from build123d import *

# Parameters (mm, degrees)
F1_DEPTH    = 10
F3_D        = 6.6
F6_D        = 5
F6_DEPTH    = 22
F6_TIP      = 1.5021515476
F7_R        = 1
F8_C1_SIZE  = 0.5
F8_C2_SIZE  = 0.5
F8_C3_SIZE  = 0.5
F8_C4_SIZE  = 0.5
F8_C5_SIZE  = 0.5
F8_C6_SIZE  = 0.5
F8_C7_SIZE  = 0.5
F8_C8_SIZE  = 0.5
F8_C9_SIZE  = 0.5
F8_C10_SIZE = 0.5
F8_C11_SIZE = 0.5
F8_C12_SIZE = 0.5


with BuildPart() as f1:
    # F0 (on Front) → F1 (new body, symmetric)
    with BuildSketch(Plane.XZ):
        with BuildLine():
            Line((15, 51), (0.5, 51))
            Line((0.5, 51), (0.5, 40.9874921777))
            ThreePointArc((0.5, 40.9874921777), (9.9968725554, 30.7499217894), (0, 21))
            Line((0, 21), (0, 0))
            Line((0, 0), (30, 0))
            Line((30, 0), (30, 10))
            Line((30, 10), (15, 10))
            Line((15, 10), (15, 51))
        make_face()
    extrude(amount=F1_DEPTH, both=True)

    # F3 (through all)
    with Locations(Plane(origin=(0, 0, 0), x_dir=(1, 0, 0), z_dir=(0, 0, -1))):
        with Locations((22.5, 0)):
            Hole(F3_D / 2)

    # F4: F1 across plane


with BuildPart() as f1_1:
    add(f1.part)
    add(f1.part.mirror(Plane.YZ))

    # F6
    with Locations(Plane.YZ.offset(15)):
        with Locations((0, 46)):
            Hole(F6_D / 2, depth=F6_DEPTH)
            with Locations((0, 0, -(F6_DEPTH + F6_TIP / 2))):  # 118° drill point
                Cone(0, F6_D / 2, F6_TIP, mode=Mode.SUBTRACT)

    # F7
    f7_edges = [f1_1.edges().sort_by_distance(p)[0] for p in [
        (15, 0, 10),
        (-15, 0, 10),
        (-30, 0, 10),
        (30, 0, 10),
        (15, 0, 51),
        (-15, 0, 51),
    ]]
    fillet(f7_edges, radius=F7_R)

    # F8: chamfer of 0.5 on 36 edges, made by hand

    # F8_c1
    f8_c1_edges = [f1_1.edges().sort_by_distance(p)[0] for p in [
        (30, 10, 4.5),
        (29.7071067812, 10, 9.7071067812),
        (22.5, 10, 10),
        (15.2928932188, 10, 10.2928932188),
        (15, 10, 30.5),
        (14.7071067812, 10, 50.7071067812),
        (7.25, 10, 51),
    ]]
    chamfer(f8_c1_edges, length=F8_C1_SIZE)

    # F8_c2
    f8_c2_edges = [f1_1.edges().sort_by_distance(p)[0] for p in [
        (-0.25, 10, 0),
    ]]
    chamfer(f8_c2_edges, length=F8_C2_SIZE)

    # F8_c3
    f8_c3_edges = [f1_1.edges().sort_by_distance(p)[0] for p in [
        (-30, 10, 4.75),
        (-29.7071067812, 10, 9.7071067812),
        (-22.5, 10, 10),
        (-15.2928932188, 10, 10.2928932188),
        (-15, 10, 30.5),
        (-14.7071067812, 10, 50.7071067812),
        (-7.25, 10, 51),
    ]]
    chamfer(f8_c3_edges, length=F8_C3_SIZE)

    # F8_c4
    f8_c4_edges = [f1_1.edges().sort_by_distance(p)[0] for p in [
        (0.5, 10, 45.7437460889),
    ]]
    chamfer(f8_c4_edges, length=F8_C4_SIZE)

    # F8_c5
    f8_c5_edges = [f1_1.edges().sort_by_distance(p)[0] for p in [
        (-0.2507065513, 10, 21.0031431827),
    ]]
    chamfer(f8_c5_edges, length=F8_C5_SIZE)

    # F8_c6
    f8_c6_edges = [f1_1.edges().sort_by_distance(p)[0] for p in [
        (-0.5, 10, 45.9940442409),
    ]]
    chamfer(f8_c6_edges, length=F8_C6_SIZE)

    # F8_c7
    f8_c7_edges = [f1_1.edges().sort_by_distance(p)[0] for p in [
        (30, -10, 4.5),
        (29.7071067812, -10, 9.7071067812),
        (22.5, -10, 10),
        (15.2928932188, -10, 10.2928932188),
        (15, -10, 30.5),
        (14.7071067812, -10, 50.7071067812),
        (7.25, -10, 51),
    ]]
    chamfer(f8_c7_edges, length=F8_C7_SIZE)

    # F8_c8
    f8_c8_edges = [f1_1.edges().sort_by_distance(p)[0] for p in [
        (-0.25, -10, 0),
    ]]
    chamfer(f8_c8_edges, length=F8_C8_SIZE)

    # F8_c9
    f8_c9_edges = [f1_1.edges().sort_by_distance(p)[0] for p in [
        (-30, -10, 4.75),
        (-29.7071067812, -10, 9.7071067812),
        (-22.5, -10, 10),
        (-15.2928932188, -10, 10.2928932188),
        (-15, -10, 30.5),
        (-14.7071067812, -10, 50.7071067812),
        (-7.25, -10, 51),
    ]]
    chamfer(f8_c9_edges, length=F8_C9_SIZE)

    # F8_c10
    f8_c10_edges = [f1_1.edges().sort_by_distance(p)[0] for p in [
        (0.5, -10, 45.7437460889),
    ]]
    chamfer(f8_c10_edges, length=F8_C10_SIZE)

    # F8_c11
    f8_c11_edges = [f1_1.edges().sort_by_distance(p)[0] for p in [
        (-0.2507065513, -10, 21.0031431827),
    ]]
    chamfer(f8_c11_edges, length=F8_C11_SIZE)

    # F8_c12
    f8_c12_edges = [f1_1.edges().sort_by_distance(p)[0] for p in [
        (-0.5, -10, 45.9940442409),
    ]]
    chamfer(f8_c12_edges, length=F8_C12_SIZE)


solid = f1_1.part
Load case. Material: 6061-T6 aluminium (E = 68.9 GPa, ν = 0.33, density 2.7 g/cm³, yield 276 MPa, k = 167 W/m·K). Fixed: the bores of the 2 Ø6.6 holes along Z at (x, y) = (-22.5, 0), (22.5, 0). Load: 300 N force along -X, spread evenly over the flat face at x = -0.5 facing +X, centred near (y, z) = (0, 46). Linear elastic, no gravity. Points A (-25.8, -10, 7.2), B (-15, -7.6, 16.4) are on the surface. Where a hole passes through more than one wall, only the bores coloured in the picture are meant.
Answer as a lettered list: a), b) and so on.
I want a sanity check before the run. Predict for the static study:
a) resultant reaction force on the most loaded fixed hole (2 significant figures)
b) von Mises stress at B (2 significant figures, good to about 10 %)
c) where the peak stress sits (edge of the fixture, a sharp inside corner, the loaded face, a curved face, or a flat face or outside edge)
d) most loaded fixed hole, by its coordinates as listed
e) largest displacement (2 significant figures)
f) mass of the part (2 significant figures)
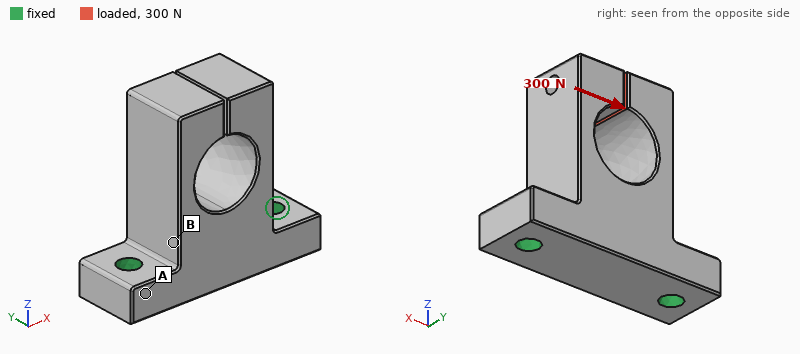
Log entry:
a) 420 N
b) 14 MPa
c) a curved face
d) (22.5, 0)
e) 0.10 mm
f) 78 g
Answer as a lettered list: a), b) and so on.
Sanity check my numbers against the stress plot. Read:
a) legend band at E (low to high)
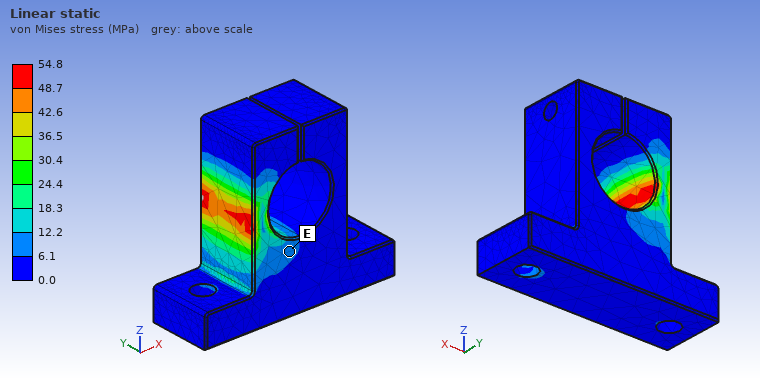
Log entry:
a) 6.1 to 12.2 MPa
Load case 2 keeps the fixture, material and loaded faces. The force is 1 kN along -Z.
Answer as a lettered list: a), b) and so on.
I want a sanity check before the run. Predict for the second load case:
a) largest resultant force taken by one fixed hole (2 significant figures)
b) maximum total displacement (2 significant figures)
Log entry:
a) 580 N
b) 0.24 mm
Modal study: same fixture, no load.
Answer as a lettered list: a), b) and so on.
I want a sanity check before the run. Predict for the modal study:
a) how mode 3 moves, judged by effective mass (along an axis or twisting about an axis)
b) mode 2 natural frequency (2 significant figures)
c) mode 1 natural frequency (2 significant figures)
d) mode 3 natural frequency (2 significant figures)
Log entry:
a) along Y
b) 3400 Hz
c) 3300 Hz
d) 3600 Hz
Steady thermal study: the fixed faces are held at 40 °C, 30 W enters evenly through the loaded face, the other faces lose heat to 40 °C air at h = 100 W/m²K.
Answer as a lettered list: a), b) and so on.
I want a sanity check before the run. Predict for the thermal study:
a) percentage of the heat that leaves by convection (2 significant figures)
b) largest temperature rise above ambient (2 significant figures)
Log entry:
a) 27 %
b) 45 K
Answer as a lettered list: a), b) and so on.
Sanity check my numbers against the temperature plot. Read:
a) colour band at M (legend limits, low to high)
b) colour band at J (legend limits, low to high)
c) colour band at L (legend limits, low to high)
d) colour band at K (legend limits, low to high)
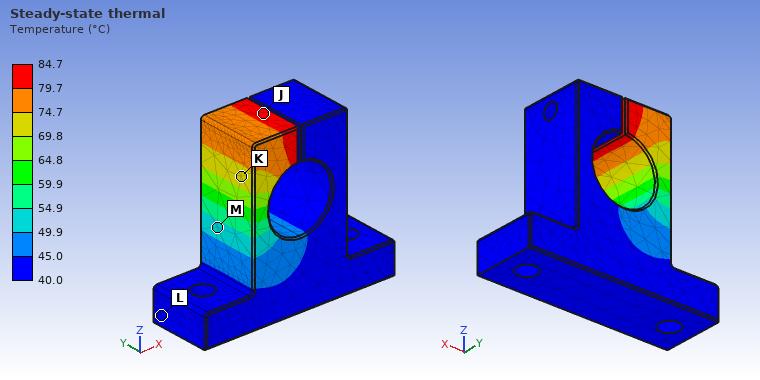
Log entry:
a) 49.9 to 54.9 °C
b) 79.7 to 84.7 °C
c) 40.0 to 45.0 °C
d) 69.8 to 74.7 °C
